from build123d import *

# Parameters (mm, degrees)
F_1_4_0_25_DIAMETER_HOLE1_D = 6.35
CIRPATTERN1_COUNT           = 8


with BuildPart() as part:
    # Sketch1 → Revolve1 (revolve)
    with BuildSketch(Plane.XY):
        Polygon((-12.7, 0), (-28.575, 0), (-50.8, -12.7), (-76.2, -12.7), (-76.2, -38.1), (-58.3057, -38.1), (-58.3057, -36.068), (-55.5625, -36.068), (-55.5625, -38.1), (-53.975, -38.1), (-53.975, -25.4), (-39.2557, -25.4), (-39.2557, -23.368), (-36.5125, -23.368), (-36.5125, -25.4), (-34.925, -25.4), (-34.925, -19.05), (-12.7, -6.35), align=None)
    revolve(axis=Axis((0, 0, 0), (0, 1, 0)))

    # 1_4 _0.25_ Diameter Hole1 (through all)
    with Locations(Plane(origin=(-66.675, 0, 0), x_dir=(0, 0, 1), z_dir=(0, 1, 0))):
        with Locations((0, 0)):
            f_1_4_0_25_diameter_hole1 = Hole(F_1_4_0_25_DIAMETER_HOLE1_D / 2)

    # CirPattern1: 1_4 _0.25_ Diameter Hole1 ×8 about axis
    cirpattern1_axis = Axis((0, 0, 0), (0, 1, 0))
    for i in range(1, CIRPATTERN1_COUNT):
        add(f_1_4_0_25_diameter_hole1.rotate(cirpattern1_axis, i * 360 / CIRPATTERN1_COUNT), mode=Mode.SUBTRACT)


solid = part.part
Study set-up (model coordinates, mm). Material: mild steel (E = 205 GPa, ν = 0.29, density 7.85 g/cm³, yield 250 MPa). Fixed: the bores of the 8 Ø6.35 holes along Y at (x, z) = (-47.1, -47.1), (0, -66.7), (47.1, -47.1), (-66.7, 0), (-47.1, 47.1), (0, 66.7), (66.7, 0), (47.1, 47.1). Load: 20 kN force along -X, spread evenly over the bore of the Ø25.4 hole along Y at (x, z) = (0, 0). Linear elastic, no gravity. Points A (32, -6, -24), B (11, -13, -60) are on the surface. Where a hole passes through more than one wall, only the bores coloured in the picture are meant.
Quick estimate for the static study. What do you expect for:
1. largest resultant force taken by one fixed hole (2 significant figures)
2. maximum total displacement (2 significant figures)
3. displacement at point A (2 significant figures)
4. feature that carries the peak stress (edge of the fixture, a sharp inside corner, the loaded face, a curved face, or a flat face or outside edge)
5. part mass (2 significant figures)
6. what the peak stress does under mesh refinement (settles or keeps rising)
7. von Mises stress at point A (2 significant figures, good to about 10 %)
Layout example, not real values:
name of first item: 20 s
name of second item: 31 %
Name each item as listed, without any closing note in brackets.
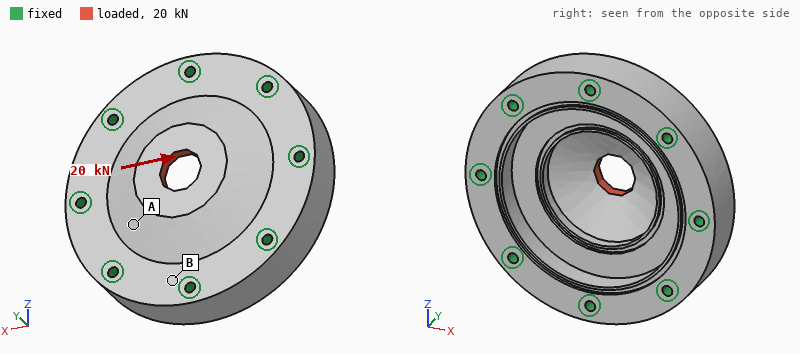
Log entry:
largest resultant force taken by one fixed hole: 4.1 kN
maximum total displacement: 8.3 µm
displacement at point A: 2.2 µm
feature that carries the peak stress: a sharp inside corner
part mass: 2.7 kg
what the peak stress does under mesh refinement: keeps rising
von Mises stress at point A: 13 MPa
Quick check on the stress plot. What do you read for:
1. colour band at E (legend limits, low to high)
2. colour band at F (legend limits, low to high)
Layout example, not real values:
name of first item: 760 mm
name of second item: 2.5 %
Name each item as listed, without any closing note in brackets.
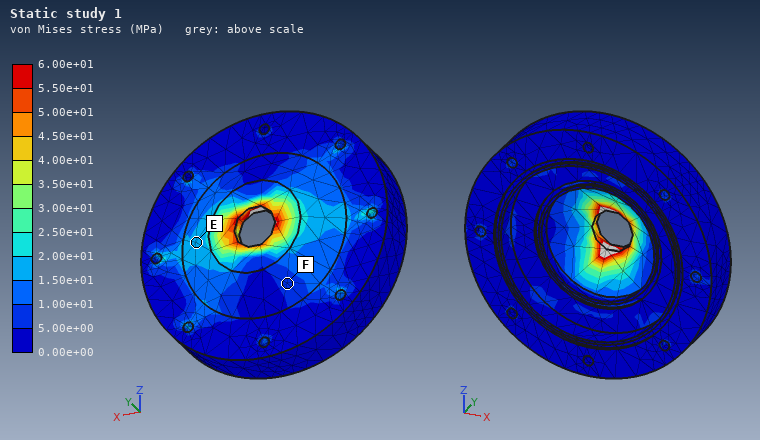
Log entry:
colour band at E: 1.50e+01 to 2.00e+01 MPa
colour band at F: 5.00e+00 to 1.00e+01 MPa
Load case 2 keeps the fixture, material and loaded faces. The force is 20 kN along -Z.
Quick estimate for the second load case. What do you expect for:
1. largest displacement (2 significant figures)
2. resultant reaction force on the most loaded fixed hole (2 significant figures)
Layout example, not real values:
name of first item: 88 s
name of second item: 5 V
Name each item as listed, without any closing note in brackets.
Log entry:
largest displacement: 8.0 µm
resultant reaction force on the most loaded fixed hole: 4.1 kN
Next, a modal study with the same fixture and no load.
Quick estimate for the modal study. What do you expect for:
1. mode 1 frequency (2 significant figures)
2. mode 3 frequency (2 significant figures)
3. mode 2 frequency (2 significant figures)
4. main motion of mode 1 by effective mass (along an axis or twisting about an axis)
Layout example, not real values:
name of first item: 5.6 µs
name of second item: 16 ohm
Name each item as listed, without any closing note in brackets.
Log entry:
mode 1 frequency: 11 kHz
mode 3 frequency: 14 kHz
mode 2 frequency: 14 kHz
main motion of mode 1 by effective mass: along Y
